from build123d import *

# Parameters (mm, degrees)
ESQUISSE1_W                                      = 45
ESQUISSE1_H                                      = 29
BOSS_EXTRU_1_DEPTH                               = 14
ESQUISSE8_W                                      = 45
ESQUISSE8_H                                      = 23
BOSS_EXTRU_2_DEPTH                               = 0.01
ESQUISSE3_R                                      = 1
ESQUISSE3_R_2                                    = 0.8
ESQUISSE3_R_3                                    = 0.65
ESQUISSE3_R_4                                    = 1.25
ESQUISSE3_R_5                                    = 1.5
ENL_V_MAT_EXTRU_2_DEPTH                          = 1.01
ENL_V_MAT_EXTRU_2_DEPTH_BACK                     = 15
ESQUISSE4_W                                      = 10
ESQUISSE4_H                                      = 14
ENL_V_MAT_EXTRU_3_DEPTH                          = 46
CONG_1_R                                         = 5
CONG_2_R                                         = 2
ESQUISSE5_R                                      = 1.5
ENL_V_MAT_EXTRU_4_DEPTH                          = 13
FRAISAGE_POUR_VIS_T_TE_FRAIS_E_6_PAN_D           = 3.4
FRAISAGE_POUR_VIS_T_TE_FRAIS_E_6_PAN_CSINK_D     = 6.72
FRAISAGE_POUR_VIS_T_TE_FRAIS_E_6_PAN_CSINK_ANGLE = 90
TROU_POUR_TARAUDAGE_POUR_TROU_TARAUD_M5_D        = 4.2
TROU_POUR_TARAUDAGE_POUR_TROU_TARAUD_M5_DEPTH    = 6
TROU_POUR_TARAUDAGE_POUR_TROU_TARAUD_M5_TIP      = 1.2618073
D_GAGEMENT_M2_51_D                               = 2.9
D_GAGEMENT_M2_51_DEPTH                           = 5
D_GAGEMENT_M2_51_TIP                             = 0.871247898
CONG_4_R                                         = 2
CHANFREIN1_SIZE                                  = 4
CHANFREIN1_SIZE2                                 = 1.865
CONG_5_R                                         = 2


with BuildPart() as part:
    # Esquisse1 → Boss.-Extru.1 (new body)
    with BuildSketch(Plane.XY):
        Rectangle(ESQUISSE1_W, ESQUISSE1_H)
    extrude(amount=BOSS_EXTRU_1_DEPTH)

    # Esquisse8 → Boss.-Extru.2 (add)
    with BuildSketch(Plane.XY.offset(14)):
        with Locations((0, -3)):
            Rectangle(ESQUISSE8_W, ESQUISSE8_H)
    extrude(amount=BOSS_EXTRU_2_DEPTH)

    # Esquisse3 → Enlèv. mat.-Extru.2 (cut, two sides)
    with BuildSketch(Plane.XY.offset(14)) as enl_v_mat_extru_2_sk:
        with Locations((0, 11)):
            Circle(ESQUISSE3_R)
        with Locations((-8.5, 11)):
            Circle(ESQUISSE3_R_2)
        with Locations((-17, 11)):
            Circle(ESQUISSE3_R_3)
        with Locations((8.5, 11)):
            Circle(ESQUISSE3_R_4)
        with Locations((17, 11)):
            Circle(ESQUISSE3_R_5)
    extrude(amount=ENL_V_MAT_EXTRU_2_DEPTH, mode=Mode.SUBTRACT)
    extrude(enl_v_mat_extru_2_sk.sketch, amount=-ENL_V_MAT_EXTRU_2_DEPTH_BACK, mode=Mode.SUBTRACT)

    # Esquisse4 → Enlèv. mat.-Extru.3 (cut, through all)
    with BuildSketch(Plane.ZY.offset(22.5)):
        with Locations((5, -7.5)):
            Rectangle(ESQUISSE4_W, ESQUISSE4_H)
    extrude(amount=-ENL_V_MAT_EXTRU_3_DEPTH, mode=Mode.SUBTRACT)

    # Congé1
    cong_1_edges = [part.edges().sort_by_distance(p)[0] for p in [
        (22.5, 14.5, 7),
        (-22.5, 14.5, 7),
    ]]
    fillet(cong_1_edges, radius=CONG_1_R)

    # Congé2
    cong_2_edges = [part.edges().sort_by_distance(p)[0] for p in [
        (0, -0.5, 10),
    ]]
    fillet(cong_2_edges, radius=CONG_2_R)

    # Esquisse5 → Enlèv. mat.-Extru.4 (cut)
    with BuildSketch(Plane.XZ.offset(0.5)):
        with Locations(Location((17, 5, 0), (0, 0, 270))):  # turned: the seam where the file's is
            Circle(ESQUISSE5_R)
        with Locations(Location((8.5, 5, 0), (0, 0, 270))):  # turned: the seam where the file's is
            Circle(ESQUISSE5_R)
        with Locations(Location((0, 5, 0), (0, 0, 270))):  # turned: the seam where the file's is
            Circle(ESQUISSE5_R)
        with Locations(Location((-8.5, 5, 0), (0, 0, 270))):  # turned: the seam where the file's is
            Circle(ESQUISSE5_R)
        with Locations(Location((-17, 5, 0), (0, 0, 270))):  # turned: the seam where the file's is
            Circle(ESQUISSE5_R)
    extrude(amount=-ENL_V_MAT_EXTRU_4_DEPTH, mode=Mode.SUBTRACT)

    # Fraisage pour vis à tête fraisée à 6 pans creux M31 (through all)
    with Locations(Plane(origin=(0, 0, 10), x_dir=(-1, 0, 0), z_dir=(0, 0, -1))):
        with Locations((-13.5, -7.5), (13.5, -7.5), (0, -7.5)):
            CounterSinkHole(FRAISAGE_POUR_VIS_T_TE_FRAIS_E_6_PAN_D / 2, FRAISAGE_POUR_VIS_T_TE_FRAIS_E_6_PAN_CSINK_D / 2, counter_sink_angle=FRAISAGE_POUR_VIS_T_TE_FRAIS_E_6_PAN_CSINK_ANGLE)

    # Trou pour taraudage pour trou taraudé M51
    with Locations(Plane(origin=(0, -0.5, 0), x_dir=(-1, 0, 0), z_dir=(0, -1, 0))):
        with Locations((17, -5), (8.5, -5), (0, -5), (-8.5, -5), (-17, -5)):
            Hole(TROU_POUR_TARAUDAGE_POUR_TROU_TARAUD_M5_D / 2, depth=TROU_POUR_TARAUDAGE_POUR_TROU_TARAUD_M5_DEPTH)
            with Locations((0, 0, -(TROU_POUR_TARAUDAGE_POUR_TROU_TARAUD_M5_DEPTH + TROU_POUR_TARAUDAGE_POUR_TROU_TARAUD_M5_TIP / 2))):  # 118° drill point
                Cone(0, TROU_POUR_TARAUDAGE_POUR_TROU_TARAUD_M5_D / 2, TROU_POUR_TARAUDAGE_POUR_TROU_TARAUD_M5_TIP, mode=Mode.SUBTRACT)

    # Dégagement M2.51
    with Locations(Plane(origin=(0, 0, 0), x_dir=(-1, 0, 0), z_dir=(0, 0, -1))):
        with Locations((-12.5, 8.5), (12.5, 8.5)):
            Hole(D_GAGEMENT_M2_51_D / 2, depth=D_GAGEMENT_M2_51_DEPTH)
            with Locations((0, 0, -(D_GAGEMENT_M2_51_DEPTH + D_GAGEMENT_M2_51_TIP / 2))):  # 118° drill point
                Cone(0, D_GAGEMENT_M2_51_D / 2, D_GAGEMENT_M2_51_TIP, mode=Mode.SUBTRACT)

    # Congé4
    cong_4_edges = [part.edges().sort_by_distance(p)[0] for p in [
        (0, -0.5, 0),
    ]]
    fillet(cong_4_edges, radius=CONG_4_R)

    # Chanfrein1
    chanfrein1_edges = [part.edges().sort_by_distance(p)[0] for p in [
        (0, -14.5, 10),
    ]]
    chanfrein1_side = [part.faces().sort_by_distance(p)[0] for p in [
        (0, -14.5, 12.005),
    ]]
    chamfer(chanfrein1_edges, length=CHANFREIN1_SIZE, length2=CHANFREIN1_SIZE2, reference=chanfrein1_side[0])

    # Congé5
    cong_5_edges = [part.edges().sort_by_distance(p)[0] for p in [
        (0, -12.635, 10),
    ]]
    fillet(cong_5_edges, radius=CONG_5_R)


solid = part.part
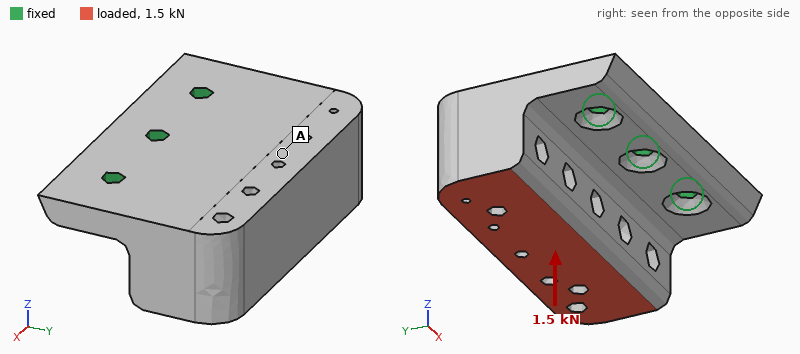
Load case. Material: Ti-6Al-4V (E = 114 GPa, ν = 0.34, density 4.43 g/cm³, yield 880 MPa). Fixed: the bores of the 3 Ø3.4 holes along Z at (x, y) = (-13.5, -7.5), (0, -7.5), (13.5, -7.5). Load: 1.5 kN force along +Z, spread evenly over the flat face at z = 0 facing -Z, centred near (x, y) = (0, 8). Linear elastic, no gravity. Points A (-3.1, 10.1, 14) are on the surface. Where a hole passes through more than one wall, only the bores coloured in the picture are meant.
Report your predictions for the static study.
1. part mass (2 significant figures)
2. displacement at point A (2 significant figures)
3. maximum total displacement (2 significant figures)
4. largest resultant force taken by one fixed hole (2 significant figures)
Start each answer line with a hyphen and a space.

- 47 g
- 0.10 mm
- 0.16 mm
- 530 N
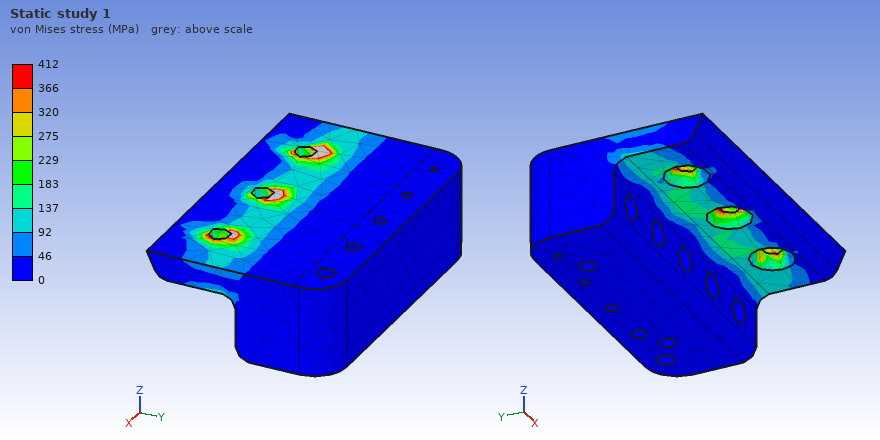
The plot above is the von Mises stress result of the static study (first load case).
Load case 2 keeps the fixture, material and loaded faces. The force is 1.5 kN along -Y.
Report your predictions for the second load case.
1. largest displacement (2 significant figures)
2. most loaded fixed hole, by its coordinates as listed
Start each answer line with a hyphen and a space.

- 0.16 mm
- (0, -7.5)
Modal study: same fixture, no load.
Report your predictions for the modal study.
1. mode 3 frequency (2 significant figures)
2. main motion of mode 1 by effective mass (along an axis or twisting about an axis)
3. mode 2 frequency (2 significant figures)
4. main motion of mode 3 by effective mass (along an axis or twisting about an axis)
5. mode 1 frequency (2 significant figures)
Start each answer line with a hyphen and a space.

- 14 kHz
- along Z
- 8600 Hz
- along X
- 3100 Hz
